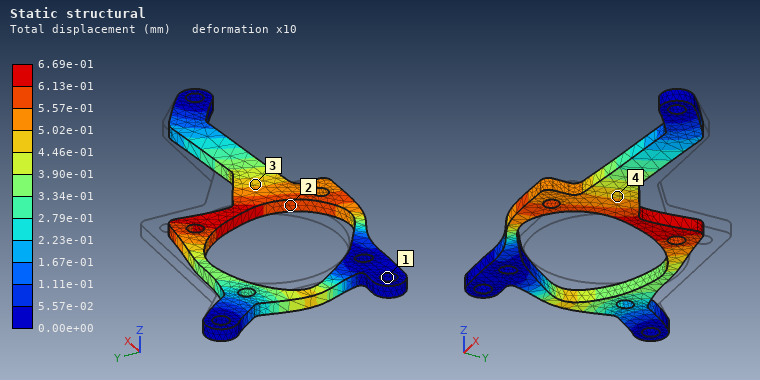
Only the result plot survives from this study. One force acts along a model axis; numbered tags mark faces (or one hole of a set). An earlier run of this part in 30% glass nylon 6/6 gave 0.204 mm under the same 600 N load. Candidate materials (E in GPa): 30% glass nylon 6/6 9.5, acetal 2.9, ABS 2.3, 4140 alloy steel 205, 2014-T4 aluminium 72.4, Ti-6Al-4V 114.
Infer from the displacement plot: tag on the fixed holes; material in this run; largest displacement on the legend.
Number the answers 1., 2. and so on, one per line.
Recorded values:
1. 1
2. acetal
3. 6.69e-01 mm
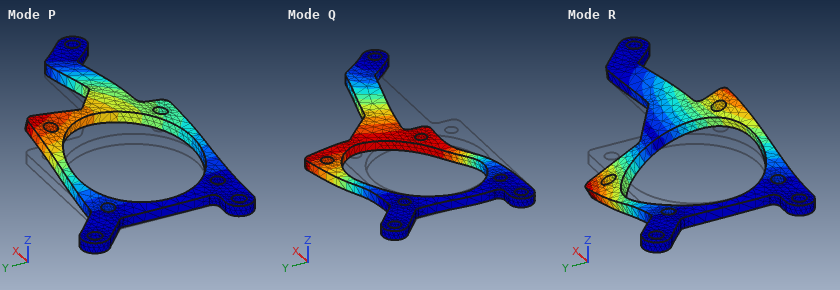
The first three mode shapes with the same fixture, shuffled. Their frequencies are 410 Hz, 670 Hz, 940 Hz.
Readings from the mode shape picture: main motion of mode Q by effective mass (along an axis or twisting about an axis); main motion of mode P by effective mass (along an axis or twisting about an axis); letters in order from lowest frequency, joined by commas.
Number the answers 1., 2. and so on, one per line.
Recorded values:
1. along Y
2. along Z
3. P, R, Q
